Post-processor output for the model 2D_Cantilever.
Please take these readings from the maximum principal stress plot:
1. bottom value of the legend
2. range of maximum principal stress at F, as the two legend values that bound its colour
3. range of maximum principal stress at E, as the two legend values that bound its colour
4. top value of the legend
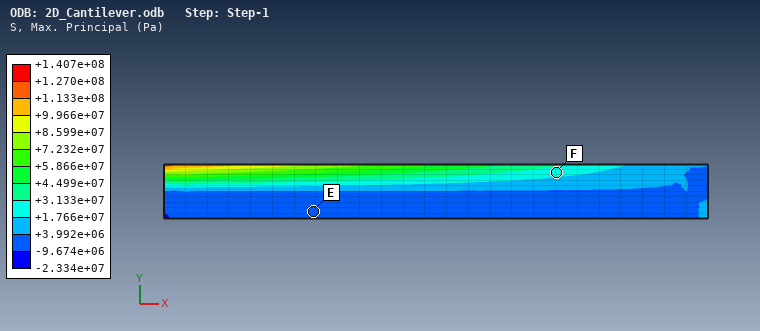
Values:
-2.334e+07 Pa
+1.766e+07 to +3.133e+07 Pa
-9.674e+06 to +3.992e+06 Pa
+1.407e+08 Pa
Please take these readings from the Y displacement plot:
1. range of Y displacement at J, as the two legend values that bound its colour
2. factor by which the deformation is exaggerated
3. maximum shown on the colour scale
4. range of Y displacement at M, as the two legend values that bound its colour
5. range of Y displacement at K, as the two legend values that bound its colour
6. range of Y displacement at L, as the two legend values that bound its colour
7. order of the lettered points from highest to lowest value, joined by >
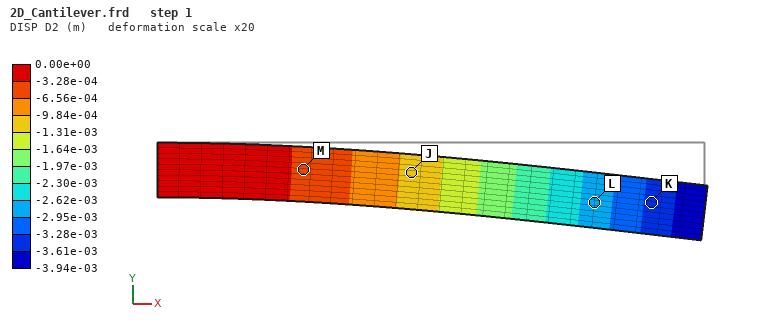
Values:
-1.31e-03 to -9.84e-04 m
20
0.00e+00 m
-6.56e-04 to -3.28e-04 m
-3.61e-03 to -3.28e-03 m
-2.95e-03 to -2.62e-03 m
M > J > L > K
